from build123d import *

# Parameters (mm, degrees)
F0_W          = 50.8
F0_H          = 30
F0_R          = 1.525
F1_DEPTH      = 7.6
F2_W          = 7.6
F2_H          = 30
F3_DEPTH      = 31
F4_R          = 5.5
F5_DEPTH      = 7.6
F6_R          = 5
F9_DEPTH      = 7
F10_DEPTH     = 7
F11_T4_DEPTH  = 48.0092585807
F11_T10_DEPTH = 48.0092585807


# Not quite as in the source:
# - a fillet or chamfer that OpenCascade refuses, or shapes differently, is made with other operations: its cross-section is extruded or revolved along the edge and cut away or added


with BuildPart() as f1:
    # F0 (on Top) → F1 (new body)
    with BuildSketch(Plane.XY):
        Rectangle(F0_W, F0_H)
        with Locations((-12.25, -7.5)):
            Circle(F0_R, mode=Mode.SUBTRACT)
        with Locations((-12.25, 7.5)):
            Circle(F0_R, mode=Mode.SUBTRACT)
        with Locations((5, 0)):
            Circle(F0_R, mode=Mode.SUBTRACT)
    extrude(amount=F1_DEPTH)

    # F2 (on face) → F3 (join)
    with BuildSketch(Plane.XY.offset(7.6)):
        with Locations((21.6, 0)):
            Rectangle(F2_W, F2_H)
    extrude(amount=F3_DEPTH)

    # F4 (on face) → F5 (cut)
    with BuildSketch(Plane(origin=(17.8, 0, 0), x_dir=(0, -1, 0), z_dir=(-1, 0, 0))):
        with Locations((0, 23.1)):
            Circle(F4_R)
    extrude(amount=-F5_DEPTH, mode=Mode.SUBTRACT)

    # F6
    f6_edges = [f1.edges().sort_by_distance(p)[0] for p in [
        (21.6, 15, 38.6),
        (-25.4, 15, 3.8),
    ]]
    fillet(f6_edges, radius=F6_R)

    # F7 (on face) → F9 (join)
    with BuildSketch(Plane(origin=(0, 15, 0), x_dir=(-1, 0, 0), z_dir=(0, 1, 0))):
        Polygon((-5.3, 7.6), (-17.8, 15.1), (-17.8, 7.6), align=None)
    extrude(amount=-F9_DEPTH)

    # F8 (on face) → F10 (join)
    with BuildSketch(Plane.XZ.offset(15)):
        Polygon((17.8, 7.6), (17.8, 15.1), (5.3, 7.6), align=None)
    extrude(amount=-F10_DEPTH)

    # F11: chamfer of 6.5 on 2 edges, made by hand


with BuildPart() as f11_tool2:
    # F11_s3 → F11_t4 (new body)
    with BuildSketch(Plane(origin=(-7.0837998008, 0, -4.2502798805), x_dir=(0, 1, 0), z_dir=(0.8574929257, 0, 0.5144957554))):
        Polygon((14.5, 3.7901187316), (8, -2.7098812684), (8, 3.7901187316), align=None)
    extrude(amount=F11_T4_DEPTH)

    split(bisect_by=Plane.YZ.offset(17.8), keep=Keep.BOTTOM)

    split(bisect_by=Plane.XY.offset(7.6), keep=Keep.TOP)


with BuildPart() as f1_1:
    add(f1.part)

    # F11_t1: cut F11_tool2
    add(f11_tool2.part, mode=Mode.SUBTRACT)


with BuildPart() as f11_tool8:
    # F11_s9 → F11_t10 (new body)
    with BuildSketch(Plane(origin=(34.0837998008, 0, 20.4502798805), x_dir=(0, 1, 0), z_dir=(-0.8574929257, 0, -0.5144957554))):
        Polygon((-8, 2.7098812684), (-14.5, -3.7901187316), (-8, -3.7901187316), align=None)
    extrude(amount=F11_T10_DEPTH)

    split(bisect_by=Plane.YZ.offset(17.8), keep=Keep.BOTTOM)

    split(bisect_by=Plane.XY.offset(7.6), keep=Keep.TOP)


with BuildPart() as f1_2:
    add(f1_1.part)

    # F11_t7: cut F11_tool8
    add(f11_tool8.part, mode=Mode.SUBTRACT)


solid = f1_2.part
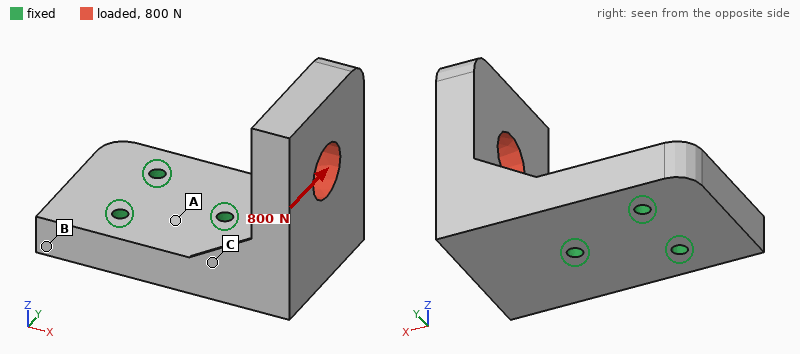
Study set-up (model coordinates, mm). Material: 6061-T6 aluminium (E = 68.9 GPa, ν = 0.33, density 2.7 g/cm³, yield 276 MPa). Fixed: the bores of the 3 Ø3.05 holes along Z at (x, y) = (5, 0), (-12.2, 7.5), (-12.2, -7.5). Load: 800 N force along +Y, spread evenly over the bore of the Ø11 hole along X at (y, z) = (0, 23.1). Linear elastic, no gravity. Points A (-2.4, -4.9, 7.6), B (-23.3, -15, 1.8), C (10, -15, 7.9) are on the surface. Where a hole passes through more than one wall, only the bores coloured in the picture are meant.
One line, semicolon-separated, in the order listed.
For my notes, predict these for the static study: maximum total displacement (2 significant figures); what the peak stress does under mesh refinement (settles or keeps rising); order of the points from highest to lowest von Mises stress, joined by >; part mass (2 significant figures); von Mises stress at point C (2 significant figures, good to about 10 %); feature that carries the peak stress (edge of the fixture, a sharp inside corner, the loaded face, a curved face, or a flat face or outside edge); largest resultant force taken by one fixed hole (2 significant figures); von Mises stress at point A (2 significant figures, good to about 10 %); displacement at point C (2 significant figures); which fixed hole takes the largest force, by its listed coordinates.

97 µm; keeps rising; C > A > B; 48 g; 32 MPa; edge of the fixture; 1.1 kN; 16 MPa; 24 µm; (5, 0)
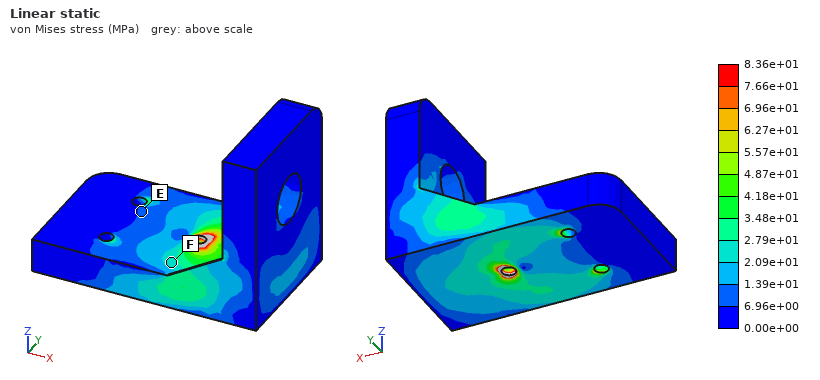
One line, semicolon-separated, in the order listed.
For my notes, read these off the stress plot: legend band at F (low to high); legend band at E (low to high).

2.09e+01 to 2.79e+01 MPa; 6.96e+00 to 1.39e+01 MPa
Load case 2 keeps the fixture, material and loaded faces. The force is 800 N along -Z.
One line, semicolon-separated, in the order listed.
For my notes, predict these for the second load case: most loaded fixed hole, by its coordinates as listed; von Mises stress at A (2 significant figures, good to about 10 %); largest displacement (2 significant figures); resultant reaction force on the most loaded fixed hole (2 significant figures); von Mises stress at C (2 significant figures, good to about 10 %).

(5, 0); 9.6 MPa; 68 µm; 1.2 kN; 16 MPa
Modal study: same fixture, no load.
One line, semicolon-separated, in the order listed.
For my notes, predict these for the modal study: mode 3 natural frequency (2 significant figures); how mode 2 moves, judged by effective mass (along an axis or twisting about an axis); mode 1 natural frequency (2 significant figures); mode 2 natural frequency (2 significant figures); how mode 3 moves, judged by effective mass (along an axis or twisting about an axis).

8700 Hz; along Y; 3200 Hz; 4000 Hz; along Z
